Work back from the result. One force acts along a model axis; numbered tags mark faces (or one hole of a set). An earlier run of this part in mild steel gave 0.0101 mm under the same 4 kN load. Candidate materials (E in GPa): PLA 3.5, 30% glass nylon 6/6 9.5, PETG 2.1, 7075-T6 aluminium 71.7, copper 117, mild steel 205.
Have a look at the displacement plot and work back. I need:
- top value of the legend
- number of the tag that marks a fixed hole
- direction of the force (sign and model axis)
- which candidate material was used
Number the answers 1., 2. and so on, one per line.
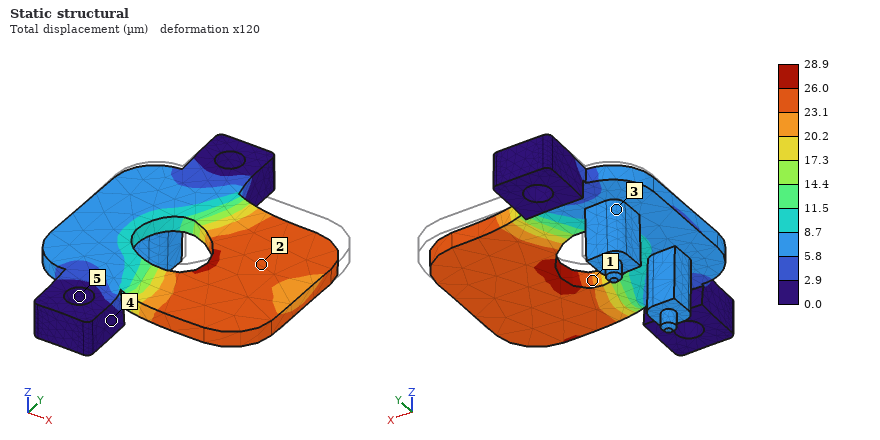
1. 28.9 µm
2. 5
3. -Y
4. 7075-T6 aluminium
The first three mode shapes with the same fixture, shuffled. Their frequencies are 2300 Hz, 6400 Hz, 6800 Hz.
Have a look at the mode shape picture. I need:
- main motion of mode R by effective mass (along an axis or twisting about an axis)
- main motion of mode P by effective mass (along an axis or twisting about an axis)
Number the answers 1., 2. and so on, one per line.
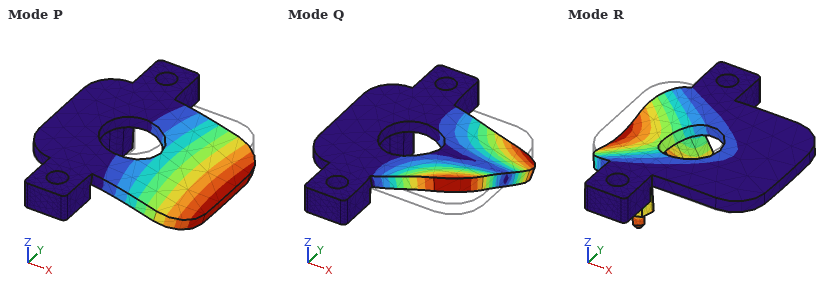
1. along Z
2. along Z
